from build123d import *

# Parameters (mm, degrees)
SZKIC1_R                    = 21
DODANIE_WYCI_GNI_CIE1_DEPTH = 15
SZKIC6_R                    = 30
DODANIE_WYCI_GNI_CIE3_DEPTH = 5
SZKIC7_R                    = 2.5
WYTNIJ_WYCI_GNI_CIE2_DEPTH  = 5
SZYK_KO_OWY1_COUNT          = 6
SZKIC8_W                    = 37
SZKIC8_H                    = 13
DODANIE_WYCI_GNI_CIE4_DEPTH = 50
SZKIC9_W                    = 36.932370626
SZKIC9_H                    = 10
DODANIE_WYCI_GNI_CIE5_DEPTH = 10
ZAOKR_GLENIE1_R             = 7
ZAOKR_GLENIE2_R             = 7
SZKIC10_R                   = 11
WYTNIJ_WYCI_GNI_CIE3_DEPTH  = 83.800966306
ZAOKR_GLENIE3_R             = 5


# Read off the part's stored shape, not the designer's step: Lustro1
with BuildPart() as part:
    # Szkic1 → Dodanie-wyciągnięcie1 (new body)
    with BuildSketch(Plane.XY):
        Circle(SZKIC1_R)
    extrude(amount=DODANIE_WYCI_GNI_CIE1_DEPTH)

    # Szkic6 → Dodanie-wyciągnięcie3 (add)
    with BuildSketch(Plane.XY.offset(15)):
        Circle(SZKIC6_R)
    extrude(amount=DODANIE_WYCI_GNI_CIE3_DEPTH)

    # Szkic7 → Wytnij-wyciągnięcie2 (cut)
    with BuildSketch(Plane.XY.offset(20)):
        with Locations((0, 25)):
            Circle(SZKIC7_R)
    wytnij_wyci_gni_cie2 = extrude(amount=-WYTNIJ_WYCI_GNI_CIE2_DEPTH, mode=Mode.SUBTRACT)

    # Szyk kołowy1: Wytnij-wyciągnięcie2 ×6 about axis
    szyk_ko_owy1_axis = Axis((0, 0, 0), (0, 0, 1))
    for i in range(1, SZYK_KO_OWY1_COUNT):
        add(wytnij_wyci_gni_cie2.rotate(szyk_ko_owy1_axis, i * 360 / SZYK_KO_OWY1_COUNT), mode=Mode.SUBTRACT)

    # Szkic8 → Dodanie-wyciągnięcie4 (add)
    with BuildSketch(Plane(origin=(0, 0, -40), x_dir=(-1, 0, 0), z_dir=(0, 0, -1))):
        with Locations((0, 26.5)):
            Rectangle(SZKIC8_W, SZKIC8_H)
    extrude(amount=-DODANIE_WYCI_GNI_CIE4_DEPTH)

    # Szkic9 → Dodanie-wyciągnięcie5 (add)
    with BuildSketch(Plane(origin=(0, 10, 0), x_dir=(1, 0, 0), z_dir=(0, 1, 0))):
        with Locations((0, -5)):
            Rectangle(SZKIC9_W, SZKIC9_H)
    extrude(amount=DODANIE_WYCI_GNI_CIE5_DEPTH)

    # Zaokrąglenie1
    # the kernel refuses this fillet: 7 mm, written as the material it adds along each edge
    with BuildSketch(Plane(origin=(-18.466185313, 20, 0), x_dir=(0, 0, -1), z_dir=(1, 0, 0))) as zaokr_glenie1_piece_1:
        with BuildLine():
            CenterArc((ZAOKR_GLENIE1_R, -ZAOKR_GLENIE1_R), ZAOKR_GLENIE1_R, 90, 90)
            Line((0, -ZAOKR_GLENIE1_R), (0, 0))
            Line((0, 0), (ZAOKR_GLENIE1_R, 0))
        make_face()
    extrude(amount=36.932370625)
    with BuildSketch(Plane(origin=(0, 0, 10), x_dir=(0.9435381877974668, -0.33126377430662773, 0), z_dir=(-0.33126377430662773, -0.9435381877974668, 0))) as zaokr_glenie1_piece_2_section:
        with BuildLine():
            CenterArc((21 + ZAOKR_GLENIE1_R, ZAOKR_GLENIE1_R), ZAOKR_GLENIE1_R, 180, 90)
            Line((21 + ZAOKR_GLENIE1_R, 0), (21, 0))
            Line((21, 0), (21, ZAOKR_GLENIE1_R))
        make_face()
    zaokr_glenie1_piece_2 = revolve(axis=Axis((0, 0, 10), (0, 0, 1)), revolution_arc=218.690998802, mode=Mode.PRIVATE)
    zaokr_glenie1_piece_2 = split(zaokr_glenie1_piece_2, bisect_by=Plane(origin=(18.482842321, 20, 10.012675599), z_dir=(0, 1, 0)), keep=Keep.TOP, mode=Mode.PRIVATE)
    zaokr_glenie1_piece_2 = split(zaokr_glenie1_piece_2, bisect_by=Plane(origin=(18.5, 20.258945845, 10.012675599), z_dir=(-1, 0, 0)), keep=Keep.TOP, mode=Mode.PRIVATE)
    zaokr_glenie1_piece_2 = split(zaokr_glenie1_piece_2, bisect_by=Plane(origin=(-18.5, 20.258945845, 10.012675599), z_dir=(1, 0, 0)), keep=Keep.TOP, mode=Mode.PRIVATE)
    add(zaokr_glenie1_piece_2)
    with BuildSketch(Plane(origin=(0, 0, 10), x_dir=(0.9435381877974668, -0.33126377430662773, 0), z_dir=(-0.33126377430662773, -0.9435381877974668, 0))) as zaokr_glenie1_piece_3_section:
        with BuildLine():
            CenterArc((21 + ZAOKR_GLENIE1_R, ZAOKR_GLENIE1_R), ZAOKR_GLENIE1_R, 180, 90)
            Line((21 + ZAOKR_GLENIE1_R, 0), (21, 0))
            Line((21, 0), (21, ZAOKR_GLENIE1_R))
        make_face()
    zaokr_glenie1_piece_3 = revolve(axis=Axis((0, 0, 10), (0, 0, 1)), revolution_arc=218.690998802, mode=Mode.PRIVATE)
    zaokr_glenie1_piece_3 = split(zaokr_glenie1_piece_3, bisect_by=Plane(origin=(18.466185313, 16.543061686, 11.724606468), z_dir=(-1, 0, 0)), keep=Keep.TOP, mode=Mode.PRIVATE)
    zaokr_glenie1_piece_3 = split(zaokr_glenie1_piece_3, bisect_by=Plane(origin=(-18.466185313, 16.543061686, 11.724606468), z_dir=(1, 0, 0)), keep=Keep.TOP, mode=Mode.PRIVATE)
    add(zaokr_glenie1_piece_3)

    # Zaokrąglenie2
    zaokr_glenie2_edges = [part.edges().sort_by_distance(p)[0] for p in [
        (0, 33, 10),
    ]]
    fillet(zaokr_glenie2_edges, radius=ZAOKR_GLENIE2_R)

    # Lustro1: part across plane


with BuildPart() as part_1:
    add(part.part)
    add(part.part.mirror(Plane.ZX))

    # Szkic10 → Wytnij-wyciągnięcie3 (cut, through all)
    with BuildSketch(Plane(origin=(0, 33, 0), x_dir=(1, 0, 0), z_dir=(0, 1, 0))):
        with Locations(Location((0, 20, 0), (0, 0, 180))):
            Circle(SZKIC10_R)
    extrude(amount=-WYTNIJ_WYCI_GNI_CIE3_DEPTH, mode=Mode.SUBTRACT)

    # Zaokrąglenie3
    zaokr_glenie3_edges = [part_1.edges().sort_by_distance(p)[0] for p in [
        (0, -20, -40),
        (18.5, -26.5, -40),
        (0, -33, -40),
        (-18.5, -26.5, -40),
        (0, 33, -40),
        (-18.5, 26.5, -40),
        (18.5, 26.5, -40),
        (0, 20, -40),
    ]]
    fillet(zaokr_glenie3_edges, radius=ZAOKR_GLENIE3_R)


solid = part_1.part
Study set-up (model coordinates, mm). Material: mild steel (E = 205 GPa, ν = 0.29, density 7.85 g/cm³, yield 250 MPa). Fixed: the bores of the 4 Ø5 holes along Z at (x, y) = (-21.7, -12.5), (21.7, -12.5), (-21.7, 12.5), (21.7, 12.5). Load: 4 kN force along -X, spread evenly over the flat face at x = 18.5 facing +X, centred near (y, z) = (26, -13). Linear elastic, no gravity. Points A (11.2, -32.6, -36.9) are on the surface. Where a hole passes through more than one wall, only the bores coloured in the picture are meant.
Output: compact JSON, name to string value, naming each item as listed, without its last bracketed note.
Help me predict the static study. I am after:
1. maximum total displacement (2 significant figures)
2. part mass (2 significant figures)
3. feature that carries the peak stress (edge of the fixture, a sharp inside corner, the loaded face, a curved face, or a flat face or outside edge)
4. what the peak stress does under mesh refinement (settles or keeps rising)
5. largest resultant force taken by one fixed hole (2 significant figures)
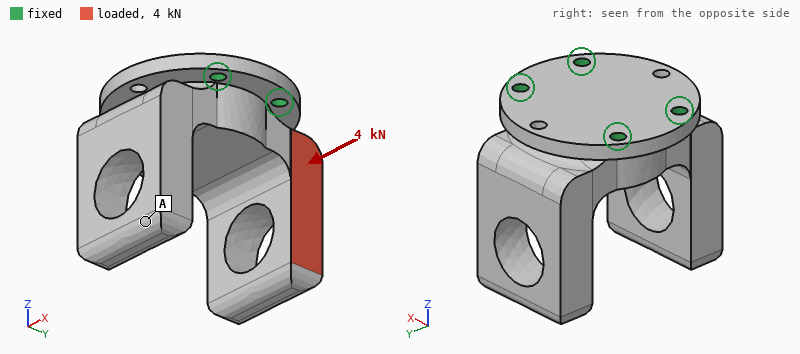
{"maximum total displacement": "36 µm", "part mass": "580 g", "feature that carries the peak stress": "edge of the fixture", "what the peak stress does under mesh refinement": "keeps rising", "largest resultant force taken by one fixed hole": "2.7 kN"}
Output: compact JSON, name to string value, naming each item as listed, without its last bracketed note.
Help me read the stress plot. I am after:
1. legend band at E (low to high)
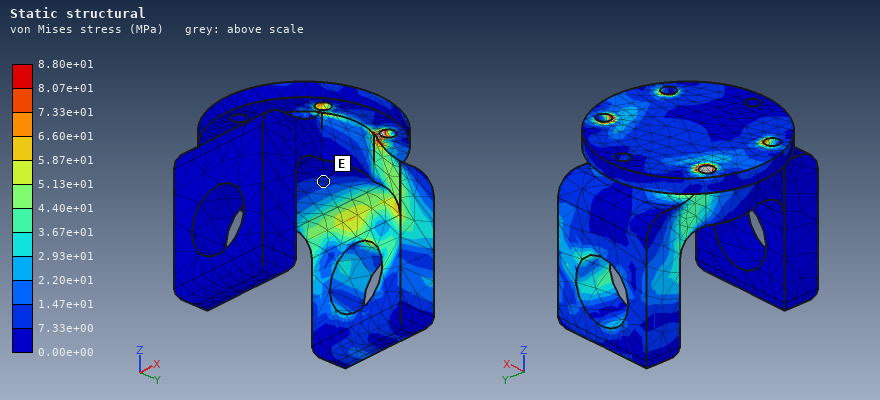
{"legend band at E": "7.33e+00 to 1.47e+01 MPa"}
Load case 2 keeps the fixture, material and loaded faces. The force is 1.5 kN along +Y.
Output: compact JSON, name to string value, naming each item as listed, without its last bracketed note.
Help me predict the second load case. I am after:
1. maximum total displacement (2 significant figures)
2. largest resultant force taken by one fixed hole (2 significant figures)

{"maximum total displacement": "38 µm", "largest resultant force taken by one fixed hole": "1.1 kN"}
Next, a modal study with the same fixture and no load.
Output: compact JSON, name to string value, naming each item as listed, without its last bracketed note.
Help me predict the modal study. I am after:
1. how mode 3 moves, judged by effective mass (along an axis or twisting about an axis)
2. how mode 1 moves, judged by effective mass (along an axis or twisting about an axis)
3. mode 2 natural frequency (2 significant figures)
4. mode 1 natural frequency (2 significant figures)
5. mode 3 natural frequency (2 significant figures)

{"how mode 3 moves, judged by effective mass": "along X", "how mode 1 moves, judged by effective mass": "along Y", "mode 2 natural frequency": "3800 Hz", "mode 1 natural frequency": "2800 Hz", "mode 3 natural frequency": "4800 Hz"}
